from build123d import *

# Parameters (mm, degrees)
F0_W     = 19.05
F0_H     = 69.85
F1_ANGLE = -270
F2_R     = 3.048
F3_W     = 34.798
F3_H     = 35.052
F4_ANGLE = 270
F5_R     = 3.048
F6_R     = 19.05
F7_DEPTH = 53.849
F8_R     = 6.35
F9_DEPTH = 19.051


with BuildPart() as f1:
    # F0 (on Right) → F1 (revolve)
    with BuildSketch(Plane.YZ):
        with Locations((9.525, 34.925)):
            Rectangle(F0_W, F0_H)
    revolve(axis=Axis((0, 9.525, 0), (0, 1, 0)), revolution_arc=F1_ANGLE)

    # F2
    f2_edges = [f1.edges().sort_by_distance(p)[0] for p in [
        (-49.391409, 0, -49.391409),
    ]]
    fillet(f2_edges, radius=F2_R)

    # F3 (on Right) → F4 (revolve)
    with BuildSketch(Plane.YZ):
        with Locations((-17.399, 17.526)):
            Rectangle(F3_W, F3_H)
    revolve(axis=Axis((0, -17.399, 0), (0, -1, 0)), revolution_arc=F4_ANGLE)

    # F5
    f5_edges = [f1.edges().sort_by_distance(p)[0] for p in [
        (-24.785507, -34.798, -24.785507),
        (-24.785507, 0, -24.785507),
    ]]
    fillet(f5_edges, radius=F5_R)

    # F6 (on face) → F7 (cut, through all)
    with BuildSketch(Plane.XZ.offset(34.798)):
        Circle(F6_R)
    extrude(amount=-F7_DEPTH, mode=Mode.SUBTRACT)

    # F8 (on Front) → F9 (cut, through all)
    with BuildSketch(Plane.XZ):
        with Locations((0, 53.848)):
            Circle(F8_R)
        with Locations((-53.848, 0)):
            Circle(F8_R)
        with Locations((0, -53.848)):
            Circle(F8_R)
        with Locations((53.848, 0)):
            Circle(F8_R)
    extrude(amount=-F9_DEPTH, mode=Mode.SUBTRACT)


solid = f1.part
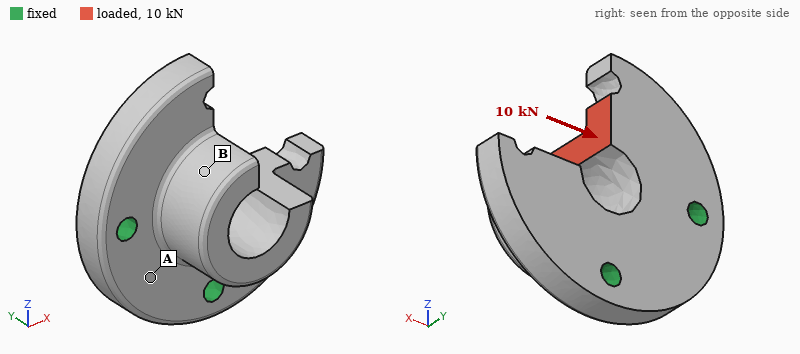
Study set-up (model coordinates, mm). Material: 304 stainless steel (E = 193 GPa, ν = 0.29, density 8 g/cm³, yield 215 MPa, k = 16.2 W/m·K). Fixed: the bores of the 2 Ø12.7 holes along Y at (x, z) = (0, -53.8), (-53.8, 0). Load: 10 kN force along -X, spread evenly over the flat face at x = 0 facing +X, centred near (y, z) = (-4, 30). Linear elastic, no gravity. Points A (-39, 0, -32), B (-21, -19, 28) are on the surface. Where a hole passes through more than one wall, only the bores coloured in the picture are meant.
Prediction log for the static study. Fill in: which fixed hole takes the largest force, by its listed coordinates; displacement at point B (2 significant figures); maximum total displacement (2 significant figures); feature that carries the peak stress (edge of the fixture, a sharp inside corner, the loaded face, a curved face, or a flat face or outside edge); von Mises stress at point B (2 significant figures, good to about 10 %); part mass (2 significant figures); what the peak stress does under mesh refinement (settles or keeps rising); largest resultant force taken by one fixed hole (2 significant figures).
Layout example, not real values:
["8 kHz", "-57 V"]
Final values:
["(-53.8, 0)", "27 µm", "47 µm", "edge of the fixture", "21 MPa", "2.1 kg", "keeps rising", "11 kN"]
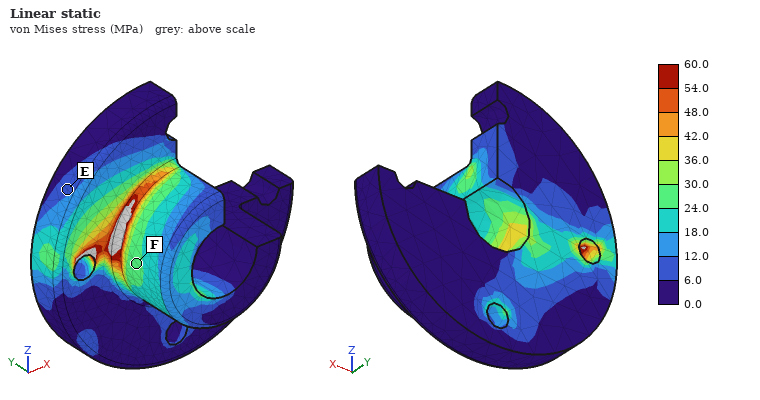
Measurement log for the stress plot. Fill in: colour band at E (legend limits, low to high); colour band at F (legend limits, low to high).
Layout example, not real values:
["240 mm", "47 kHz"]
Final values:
["6.0 to 12.0 MPa", "24.0 to 30.0 MPa"]
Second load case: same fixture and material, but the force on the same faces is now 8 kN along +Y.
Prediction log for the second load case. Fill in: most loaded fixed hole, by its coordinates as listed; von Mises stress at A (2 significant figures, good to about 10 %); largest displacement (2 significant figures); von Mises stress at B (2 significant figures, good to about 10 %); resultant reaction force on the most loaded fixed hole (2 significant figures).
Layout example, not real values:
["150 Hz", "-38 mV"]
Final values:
["(-53.8, 0)", "11 MPa", "97 µm", "13 MPa", "7.0 kN"]
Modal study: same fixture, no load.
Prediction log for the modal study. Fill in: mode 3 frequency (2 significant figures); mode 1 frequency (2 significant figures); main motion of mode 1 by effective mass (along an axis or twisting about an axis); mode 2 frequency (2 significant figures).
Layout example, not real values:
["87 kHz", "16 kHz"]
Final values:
["4700 Hz", "2400 Hz", "along Y", "3300 Hz"]
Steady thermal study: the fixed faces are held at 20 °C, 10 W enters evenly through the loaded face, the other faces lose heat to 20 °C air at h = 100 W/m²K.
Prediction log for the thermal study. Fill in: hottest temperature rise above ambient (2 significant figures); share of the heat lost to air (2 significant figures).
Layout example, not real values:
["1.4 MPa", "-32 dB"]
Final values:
["17 K", "80 %"]
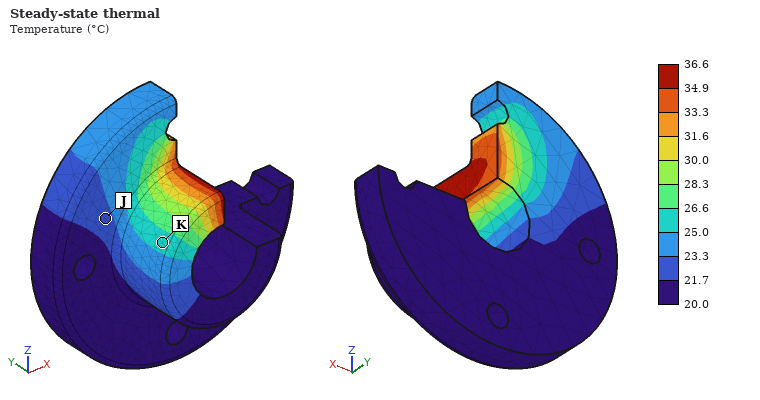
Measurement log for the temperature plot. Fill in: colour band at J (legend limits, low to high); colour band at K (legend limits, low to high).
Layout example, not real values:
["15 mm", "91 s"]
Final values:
["21.7 to 23.3 °C", "25.0 to 26.6 °C"]
